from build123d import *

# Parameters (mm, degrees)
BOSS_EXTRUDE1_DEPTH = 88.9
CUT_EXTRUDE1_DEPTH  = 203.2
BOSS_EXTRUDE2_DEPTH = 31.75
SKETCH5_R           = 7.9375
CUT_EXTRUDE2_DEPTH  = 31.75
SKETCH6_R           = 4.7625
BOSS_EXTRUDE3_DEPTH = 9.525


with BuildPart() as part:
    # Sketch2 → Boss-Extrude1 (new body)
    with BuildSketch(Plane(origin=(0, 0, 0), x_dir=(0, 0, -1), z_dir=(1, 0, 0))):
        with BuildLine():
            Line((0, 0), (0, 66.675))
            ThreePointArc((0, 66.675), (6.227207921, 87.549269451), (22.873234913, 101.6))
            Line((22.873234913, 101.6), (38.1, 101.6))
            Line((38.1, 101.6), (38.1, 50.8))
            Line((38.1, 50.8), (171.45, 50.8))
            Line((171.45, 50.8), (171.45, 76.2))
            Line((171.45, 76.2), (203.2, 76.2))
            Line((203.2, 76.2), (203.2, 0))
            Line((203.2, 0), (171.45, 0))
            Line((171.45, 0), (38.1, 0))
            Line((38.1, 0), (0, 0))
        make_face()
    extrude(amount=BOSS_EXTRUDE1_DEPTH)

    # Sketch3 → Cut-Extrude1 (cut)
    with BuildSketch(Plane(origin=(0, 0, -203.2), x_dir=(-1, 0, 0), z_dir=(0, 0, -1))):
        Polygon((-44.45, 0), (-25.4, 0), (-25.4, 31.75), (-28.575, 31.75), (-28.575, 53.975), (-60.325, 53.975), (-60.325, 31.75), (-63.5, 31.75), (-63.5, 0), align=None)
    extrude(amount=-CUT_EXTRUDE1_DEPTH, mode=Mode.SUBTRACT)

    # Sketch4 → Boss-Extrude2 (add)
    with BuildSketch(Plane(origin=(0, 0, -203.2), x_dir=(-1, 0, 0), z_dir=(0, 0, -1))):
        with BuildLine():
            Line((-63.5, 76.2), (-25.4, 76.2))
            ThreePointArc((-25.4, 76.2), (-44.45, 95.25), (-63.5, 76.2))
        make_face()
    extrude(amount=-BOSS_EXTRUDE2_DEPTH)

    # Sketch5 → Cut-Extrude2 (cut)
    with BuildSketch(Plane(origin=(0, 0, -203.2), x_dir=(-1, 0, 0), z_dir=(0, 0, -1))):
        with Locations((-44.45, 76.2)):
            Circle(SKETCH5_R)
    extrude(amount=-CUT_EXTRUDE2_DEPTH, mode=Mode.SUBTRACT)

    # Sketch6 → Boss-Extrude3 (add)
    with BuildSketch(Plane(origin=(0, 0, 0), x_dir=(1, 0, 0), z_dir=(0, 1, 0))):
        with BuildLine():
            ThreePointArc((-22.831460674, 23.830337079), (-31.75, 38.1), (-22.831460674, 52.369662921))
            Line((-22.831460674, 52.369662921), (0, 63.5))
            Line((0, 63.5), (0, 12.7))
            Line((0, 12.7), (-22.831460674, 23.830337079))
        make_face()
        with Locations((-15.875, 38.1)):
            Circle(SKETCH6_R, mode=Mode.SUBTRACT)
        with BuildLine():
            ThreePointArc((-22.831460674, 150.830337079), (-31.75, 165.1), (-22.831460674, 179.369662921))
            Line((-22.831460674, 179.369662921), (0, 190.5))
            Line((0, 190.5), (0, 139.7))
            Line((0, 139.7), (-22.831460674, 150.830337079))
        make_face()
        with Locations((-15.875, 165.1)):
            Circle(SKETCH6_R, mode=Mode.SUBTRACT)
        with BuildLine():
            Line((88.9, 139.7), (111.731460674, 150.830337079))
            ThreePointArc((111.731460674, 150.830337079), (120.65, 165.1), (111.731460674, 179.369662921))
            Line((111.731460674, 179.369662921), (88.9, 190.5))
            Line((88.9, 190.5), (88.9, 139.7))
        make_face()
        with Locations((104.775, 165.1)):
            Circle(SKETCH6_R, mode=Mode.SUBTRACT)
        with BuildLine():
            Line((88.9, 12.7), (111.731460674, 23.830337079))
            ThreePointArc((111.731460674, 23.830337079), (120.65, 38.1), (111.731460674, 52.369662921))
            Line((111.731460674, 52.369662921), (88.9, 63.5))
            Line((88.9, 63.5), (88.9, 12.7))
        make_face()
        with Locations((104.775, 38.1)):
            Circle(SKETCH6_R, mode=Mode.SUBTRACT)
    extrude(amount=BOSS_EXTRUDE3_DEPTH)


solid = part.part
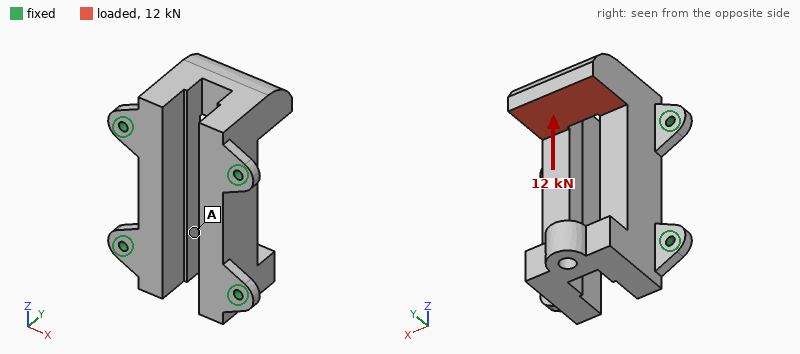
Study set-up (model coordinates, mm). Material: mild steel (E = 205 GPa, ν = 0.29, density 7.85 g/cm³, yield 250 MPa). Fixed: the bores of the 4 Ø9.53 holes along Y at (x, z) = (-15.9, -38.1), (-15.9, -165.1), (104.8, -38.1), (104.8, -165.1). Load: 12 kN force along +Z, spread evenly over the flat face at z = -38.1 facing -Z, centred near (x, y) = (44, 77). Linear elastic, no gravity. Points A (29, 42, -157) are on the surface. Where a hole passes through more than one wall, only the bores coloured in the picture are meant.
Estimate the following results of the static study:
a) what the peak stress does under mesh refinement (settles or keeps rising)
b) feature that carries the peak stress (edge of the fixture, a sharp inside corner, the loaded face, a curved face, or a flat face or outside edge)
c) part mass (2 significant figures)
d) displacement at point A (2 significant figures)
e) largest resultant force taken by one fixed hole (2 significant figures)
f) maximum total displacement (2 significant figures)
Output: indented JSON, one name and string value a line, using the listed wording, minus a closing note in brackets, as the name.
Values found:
{
  "what the peak stress does under mesh refinement": "keeps rising",
  "feature that carries the peak stress": "edge of the fixture",
  "part mass": "6.4 kg",
  "displacement at point A": "11 µm",
  "largest resultant force taken by one fixed hole": "5.5 kN",
  "maximum total displacement": "50 µm"
}
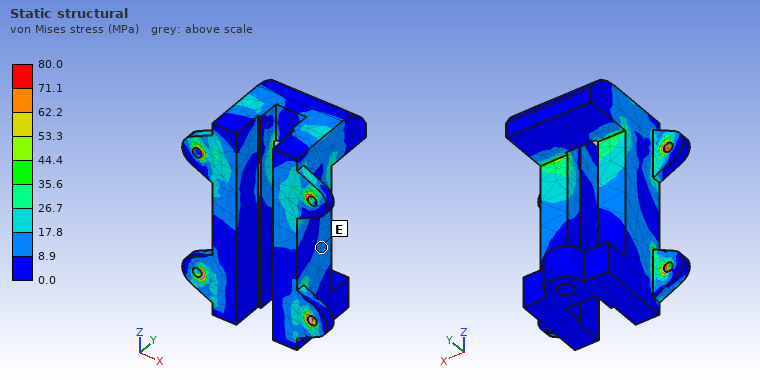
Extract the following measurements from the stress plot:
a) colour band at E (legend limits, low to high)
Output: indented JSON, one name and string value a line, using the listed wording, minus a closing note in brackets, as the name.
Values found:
{
  "colour band at E": "8.9 to 17.8 MPa"
}
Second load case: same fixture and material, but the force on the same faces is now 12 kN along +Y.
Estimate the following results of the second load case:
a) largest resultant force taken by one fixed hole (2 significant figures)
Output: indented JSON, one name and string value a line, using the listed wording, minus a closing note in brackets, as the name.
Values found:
{
  "largest resultant force taken by one fixed hole": "6.4 kN"
}
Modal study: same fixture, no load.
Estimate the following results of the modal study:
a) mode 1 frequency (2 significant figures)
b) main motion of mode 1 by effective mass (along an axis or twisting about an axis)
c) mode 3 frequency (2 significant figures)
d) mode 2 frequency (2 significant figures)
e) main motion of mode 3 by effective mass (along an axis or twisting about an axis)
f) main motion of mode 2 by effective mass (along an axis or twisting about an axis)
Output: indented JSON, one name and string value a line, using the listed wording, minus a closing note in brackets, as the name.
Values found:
{
  "mode 1 frequency": "1900 Hz",
  "main motion of mode 1 by effective mass": "along Z",
  "mode 3 frequency": "2600 Hz",
  "mode 2 frequency": "2400 Hz",
  "main motion of mode 3 by effective mass": "along Y",
  "main motion of mode 2 by effective mass": "along X"
}
